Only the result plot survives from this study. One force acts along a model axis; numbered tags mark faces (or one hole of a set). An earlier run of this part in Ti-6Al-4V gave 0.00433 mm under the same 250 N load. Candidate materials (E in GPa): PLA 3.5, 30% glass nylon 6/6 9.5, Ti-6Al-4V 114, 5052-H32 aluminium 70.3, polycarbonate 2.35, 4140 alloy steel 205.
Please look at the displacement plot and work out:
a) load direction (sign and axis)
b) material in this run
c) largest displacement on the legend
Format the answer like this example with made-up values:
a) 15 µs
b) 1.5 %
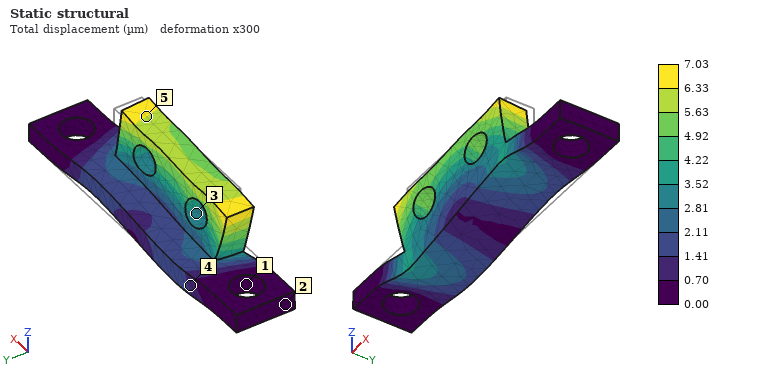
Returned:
a) -X
b) 5052-H32 aluminium
c) 7.03 µm
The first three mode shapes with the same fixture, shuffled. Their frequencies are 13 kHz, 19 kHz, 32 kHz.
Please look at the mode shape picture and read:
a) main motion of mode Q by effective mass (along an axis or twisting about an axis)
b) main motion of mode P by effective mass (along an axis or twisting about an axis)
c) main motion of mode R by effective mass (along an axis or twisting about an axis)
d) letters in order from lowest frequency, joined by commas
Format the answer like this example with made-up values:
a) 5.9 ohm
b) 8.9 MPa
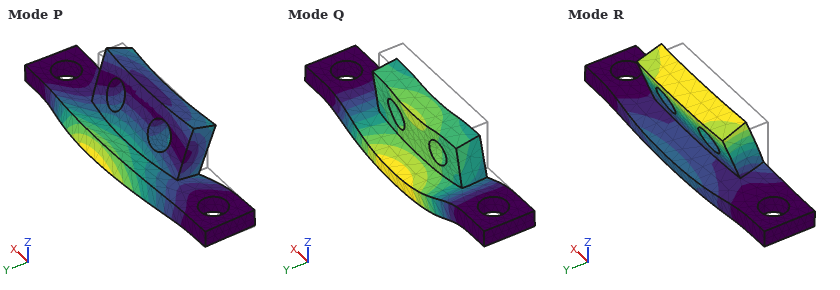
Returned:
a) along Z
b) along Y
c) along Y
d) R, Q, P
